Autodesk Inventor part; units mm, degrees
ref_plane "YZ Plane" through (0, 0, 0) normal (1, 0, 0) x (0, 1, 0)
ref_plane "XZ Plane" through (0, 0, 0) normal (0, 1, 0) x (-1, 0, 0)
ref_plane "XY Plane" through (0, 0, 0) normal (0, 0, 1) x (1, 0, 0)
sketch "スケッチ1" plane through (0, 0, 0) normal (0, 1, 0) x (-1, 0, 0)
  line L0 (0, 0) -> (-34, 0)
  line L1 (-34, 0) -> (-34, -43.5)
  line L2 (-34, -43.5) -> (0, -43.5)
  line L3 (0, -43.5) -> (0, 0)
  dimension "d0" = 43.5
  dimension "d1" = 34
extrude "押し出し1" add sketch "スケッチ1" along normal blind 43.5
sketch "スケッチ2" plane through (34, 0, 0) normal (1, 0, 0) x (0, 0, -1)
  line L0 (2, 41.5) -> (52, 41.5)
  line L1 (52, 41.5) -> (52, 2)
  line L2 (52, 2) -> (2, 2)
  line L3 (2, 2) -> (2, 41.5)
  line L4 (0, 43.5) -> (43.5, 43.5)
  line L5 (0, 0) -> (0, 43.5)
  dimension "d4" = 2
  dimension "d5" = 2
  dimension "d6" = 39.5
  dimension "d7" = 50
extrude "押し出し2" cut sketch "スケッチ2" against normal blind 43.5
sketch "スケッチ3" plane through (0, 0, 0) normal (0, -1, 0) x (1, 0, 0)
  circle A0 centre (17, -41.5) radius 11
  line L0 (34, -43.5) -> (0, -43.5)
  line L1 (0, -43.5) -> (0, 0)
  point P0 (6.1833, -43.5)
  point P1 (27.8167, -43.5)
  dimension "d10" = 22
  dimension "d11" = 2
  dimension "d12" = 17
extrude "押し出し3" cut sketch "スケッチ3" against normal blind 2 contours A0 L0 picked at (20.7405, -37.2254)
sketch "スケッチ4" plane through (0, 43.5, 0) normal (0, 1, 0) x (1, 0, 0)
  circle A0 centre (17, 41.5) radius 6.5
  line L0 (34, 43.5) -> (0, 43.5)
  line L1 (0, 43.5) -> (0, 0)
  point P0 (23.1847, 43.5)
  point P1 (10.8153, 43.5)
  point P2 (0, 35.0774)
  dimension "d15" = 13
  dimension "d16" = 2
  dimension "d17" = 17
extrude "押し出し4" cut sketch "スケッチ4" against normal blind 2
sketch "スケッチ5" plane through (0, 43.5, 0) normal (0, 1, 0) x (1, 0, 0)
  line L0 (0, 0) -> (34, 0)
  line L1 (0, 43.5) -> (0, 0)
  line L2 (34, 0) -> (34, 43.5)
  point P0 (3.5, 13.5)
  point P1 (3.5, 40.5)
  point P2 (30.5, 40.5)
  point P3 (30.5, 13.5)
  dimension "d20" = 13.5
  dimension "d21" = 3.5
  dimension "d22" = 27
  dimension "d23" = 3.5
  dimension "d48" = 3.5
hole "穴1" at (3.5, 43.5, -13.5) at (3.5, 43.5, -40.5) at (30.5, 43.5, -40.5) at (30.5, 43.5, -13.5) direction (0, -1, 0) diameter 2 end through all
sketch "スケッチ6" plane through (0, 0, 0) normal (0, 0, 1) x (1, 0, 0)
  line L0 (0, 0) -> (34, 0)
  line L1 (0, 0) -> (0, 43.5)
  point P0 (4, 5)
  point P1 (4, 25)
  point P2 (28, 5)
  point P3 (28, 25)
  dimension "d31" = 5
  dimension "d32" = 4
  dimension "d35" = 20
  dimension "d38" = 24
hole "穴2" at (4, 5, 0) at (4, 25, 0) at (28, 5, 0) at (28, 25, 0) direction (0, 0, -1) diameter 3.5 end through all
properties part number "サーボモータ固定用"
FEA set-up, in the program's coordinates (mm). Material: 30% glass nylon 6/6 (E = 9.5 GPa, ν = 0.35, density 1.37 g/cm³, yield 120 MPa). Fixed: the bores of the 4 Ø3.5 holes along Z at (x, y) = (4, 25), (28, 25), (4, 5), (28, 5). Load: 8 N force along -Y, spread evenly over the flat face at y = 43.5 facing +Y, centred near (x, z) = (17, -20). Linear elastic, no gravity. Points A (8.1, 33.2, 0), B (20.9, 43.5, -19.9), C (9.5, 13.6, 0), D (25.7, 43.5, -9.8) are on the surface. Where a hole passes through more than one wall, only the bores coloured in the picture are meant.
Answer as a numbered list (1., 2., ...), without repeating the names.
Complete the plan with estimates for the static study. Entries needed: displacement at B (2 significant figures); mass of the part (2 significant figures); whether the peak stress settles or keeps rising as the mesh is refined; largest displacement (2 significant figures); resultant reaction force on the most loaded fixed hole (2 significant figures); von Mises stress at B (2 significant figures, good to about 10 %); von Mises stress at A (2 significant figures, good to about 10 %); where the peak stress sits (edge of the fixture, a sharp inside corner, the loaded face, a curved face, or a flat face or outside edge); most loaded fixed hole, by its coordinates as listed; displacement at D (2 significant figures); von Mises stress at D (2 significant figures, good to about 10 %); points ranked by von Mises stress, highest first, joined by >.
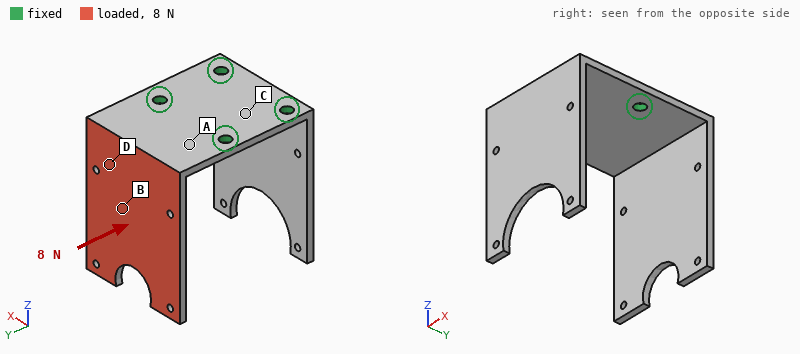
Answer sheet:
1. 0.32 mm
2. 11 g
3. keeps rising
4. 0.77 mm
5. 3.8 N
6. 1.7 MPa
7. 5.9 MPa
8. edge of the fixture
9. (28, 25)
10. 0.17 mm
11. 3.8 MPa
12. A > D > B > C
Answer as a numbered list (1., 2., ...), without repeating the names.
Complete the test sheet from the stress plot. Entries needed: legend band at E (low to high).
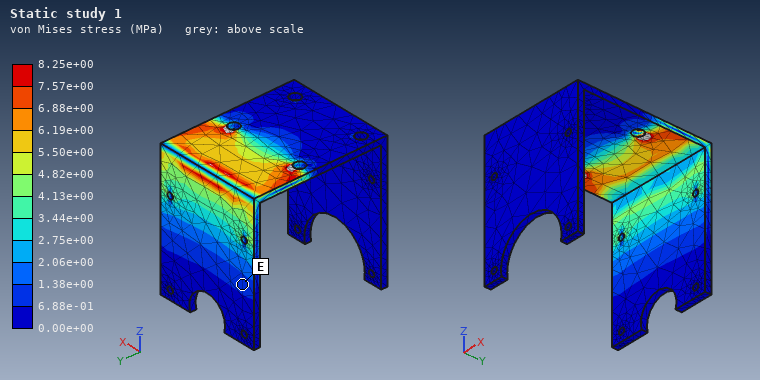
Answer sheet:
1. 6.88e-01 to 1.38e+00 MPa
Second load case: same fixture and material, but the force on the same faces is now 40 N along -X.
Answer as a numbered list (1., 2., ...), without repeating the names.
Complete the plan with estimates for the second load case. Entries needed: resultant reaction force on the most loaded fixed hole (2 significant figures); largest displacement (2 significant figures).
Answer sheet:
1. 46 N
2. 0.72 mm
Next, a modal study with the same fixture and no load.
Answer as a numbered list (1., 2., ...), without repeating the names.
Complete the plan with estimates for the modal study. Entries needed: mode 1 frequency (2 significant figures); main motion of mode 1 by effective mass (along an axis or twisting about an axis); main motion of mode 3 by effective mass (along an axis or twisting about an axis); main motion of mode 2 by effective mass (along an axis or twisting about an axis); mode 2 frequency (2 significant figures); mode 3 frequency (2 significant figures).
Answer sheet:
1. 330 Hz
2. along Y
3. along X
4. along Y
5. 570 Hz
6. 710 Hz
